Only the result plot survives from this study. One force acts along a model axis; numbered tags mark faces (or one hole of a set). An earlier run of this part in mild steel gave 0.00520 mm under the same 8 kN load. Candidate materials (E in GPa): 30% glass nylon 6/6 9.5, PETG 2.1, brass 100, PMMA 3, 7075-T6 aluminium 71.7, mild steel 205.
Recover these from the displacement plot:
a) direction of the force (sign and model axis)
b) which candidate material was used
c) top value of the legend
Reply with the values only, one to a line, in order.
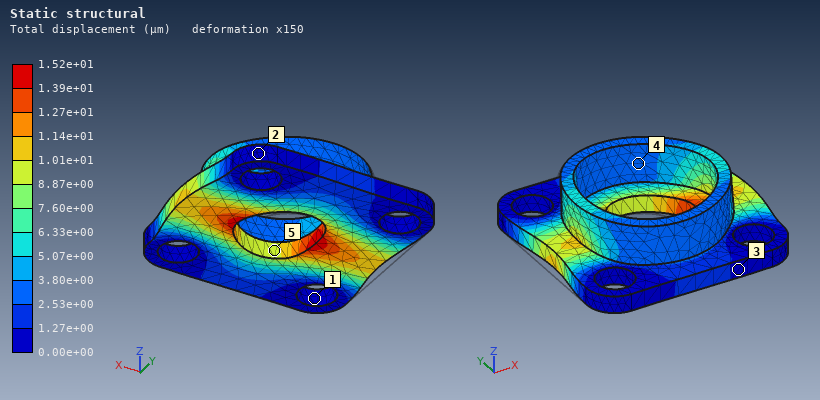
+X
7075-T6 aluminium
1.52e+01 µm
